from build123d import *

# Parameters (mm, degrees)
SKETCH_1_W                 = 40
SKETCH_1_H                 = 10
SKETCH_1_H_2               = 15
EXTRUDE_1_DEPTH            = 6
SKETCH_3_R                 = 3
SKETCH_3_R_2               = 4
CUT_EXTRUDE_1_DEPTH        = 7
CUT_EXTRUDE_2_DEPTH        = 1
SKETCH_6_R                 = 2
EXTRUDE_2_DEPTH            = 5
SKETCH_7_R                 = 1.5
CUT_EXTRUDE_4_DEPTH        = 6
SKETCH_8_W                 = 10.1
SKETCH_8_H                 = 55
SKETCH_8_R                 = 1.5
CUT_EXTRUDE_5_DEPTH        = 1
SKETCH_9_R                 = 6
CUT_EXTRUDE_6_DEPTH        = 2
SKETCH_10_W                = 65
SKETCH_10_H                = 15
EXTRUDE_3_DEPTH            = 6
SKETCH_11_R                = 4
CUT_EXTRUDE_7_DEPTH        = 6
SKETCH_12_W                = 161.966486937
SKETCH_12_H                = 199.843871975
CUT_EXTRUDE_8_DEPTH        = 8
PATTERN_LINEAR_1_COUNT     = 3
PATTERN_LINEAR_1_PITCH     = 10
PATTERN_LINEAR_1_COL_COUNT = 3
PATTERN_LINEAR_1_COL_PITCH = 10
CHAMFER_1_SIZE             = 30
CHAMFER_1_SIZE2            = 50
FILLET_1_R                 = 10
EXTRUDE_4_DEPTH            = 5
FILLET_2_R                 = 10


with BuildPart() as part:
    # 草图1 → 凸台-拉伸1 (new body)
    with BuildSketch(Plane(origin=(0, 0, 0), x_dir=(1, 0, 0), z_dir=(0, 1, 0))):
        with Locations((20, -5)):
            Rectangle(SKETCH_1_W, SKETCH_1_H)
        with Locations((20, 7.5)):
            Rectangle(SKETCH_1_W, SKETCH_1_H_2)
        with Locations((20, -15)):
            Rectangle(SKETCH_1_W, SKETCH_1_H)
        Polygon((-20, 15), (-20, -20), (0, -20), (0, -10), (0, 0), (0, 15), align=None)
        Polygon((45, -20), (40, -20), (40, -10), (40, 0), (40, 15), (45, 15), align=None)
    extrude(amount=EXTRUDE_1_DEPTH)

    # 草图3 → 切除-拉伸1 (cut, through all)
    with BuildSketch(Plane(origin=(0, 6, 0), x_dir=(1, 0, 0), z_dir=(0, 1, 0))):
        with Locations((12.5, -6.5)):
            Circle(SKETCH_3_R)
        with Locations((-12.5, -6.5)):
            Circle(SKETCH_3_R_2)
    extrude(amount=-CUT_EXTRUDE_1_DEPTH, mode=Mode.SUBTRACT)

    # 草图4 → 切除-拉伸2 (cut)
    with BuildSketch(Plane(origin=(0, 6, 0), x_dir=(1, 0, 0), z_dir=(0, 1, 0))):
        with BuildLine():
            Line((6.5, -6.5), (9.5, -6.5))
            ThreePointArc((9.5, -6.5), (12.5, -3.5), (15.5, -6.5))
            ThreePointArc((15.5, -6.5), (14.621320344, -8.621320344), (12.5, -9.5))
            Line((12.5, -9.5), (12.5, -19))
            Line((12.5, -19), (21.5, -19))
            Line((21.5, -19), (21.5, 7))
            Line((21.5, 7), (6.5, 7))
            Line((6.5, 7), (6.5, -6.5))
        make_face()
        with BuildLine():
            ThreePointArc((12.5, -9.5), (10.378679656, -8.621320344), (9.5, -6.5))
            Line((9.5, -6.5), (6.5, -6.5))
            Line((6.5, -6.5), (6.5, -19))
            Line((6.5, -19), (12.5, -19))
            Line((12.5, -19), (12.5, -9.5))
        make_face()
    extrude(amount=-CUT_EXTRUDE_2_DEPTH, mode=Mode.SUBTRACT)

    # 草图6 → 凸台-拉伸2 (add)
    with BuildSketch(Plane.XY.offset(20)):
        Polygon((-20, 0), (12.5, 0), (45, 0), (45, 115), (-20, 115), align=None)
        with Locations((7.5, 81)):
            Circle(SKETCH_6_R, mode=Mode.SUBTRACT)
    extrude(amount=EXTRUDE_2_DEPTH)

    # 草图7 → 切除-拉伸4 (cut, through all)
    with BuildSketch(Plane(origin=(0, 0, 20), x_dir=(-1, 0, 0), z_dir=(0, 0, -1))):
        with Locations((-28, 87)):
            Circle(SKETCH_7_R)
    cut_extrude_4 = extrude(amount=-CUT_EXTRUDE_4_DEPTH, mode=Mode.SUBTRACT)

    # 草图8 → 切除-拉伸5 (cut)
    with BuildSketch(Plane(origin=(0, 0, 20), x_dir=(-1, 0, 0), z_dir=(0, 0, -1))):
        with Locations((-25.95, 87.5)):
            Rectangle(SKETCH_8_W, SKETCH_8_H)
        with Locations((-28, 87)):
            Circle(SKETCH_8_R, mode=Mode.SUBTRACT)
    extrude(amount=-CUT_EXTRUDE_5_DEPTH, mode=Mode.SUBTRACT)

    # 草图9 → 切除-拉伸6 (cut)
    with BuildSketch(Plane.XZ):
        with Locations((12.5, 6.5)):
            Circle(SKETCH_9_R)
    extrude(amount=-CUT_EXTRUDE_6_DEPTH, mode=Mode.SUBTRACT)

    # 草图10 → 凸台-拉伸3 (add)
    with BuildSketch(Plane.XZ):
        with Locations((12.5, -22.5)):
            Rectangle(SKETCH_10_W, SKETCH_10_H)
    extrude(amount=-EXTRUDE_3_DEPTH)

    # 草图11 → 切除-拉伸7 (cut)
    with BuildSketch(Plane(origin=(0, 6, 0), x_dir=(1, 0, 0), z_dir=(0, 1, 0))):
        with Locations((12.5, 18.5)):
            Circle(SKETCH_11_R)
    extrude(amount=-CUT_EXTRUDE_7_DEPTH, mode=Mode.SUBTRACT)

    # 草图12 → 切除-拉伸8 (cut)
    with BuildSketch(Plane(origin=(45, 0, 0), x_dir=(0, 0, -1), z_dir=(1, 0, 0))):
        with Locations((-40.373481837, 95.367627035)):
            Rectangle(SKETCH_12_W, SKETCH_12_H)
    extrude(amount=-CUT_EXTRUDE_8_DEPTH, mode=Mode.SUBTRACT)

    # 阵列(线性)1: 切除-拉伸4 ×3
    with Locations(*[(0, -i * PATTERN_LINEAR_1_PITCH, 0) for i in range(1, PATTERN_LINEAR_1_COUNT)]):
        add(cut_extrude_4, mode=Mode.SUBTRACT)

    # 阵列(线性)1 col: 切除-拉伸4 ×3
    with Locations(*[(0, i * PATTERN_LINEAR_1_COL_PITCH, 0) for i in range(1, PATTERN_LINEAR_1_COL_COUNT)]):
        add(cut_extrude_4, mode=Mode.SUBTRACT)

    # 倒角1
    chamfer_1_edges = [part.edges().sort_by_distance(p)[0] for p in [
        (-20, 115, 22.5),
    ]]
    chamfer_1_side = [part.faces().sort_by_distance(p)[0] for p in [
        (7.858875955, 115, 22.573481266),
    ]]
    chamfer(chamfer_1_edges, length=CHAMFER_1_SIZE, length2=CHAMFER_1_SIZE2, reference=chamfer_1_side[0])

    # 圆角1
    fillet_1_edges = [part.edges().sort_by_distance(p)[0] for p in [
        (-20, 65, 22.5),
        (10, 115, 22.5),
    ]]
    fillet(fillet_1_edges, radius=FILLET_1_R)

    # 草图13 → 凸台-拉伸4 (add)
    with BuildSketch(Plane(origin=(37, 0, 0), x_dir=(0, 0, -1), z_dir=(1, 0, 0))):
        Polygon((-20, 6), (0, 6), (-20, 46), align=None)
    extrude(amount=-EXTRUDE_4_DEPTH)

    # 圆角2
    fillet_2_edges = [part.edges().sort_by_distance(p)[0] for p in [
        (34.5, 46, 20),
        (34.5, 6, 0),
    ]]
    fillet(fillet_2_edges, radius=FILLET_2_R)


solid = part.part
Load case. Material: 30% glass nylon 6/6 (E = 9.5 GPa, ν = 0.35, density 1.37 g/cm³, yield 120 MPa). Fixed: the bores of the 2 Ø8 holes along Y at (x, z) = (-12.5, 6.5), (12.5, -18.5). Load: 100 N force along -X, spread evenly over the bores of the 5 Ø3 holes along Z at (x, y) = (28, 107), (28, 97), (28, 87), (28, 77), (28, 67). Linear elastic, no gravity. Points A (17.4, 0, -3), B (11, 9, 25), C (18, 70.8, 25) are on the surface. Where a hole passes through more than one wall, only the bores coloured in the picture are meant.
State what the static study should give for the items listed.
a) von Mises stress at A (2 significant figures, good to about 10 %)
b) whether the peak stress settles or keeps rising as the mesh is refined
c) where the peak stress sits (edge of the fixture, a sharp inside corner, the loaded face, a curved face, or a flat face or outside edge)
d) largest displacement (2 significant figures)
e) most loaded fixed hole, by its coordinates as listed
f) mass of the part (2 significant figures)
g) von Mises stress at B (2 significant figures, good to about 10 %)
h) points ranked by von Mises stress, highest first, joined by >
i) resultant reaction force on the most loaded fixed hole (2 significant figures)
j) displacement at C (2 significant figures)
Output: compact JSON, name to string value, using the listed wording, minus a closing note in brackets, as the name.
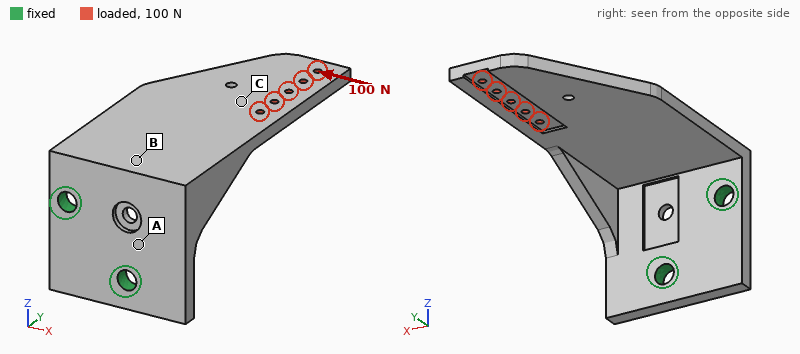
{"von Mises stress at A": "13 MPa", "whether the peak stress settles or keeps rising as the mesh is refined": "keeps rising", "where the peak stress sits": "edge of the fixture", "largest displacement": "1.5 mm", "most loaded fixed hole, by its coordinates as listed": "(-12.5, 6.5)", "mass of the part": "63 g", "von Mises stress at B": "5.8 MPa", "points ranked by von Mises stress, highest first, joined by >": "A > B > C", "resultant reaction force on the most loaded fixed hole": "150 N", "displacement at C": "0.88 mm"}
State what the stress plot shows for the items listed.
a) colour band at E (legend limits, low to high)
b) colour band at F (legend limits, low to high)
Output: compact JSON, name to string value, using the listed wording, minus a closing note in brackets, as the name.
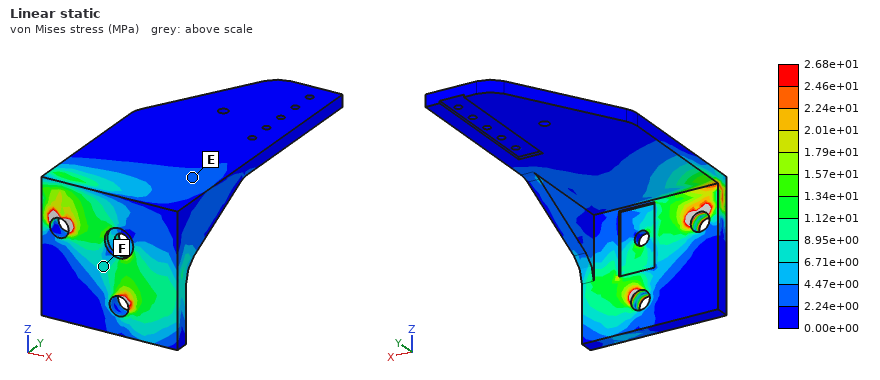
{"colour band at E": "2.24e+00 to 4.47e+00 MPa", "colour band at F": "6.71e+00 to 8.95e+00 MPa"}
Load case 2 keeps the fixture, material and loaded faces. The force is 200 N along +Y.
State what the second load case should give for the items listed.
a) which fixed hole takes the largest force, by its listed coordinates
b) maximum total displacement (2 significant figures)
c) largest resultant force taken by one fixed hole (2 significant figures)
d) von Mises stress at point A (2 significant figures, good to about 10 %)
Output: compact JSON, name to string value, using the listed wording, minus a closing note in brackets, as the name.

{"which fixed hole takes the largest force, by its listed coordinates": "(-12.5, 6.5)", "maximum total displacement": "1.7 mm", "largest resultant force taken by one fixed hole": "130 N", "von Mises stress at point A": "13 MPa"}
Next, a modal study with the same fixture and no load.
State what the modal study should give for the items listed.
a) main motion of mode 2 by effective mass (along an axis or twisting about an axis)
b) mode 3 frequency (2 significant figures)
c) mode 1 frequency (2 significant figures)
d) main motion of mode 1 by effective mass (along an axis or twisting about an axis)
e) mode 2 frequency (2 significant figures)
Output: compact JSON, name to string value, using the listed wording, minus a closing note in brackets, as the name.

{"main motion of mode 2 by effective mass": "along X", "mode 3 frequency": "870 Hz", "mode 1 frequency": "210 Hz", "main motion of mode 1 by effective mass": "along Z", "mode 2 frequency": "450 Hz"}
